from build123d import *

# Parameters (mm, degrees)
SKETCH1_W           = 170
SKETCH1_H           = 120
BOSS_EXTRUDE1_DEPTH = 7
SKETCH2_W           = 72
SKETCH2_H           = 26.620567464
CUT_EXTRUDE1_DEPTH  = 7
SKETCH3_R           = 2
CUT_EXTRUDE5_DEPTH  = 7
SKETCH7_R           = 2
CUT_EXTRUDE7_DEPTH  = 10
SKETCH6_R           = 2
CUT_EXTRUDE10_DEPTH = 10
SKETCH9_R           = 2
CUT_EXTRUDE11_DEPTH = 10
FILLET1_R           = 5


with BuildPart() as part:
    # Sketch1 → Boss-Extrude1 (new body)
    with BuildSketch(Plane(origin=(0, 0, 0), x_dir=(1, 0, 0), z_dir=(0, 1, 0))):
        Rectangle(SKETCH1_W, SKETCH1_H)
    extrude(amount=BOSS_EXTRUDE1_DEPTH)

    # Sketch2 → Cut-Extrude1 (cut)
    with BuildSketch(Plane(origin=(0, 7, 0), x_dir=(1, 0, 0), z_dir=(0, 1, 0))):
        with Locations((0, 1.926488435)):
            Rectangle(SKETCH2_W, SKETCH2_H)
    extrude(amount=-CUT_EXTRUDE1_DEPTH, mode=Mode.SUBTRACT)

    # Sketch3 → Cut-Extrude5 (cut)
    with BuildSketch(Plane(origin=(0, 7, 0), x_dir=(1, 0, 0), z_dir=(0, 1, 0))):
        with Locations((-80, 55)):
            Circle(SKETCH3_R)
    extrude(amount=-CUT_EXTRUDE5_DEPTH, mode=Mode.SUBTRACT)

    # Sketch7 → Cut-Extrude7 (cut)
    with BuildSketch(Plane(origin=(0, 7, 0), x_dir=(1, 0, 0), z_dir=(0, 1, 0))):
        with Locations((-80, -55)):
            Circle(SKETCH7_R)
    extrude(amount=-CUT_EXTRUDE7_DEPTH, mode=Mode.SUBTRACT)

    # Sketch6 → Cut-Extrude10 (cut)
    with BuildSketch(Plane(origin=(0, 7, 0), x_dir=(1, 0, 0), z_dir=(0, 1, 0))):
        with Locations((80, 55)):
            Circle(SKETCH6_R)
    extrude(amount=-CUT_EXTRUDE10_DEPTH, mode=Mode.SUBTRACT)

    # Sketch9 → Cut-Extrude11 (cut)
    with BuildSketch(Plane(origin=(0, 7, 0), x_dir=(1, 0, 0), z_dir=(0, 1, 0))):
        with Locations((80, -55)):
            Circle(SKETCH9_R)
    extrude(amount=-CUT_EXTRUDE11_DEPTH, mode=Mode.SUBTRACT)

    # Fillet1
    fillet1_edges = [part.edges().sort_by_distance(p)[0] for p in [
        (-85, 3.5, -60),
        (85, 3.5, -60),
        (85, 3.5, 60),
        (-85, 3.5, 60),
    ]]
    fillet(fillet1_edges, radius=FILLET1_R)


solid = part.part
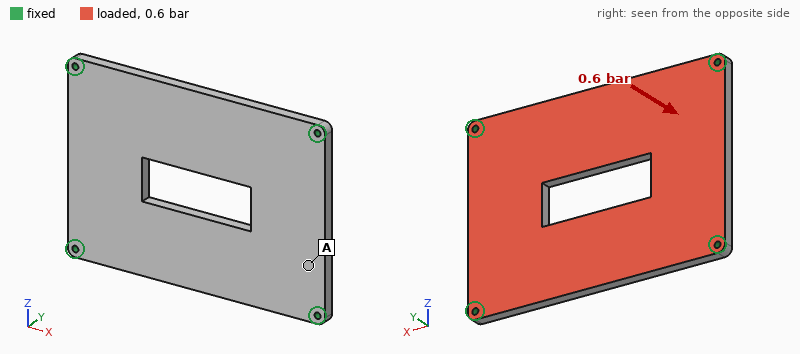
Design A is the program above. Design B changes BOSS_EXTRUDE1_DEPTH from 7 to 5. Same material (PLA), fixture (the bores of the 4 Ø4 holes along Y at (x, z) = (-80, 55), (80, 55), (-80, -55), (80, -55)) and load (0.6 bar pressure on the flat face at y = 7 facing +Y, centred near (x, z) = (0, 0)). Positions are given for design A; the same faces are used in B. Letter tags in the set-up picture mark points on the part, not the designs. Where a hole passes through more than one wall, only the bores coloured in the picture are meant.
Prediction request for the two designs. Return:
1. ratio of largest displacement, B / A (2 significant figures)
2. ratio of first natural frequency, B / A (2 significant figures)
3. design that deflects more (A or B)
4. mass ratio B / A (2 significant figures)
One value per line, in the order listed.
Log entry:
2.6
0.74
B
0.71
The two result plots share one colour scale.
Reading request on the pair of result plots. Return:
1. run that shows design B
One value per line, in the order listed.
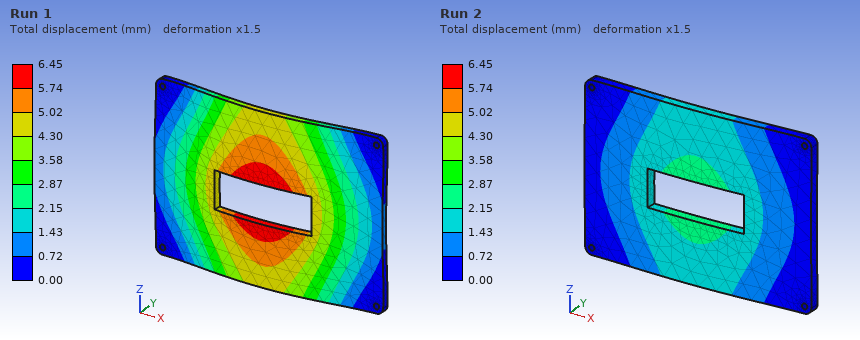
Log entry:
Run 1
